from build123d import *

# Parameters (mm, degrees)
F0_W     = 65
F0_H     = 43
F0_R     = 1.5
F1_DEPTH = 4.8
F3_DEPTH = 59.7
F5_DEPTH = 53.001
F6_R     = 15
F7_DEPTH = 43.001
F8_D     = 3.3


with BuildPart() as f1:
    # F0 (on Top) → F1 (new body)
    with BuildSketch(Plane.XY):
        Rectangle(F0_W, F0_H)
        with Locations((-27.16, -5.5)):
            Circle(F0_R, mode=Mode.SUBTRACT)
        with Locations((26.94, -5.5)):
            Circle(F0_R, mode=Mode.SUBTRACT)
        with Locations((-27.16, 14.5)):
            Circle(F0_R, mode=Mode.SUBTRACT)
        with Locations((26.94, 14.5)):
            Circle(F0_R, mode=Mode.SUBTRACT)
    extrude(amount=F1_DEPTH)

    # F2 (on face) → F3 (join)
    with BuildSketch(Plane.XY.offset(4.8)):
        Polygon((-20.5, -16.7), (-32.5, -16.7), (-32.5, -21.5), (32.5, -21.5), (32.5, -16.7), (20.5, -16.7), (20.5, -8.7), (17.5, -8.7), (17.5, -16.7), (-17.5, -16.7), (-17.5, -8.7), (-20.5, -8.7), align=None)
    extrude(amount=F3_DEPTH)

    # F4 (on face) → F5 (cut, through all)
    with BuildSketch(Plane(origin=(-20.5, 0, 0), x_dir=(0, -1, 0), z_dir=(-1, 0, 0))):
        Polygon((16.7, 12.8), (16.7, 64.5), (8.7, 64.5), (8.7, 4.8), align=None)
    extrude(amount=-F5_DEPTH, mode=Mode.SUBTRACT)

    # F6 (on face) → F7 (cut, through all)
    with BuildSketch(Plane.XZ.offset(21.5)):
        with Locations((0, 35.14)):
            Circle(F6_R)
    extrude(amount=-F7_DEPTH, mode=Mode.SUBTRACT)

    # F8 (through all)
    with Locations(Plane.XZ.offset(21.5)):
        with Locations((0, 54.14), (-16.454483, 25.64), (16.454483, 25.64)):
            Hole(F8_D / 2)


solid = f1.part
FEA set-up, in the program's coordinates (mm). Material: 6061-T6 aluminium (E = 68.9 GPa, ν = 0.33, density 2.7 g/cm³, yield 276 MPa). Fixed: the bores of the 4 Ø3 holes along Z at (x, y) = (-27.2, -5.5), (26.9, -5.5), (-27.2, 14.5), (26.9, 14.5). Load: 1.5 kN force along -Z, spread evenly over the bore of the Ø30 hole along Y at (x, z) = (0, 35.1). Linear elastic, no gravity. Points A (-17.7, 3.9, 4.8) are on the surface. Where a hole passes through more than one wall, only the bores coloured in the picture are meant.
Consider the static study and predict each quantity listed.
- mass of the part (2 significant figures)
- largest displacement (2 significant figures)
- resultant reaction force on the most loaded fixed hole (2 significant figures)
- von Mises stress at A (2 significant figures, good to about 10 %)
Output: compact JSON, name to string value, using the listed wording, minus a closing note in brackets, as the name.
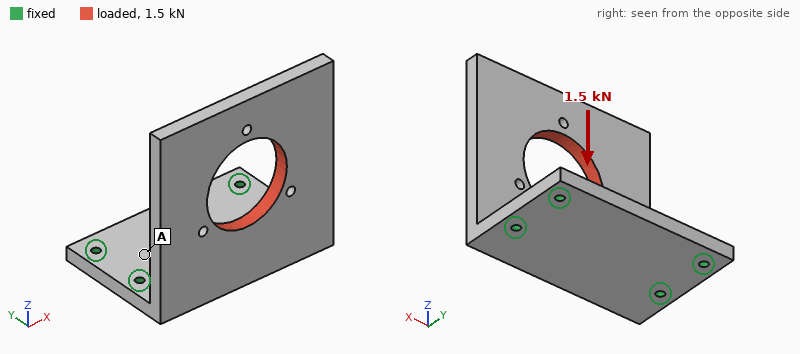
{"mass of the part": "77 g", "largest displacement": "0.28 mm", "resultant reaction force on the most loaded fixed hole": "960 N", "von Mises stress at A": "20 MPa"}
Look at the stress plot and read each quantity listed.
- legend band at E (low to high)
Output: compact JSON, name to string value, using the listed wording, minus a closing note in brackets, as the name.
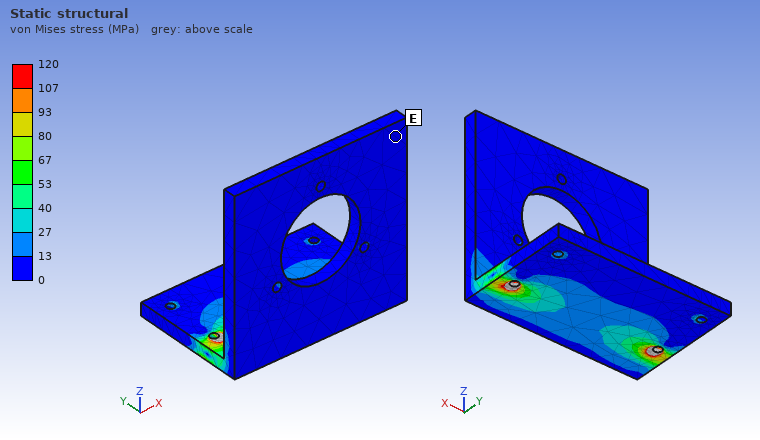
{"legend band at E": "0 to 13 MPa"}
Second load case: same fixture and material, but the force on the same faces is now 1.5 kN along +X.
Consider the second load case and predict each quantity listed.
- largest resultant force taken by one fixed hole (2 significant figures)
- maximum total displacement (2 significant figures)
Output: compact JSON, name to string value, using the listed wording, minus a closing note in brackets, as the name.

{"largest resultant force taken by one fixed hole": "1.2 kN", "maximum total displacement": "0.17 mm"}
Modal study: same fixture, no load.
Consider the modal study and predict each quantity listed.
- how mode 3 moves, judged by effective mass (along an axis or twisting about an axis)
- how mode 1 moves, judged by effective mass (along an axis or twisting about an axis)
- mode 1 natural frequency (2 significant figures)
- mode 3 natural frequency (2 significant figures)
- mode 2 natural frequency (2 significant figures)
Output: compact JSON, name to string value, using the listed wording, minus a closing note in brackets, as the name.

{"how mode 3 moves, judged by effective mass": "along X", "how mode 1 moves, judged by effective mass": "along Y", "mode 1 natural frequency": "800 Hz", "mode 3 natural frequency": "3100 Hz", "mode 2 natural frequency": "1900 Hz"}
